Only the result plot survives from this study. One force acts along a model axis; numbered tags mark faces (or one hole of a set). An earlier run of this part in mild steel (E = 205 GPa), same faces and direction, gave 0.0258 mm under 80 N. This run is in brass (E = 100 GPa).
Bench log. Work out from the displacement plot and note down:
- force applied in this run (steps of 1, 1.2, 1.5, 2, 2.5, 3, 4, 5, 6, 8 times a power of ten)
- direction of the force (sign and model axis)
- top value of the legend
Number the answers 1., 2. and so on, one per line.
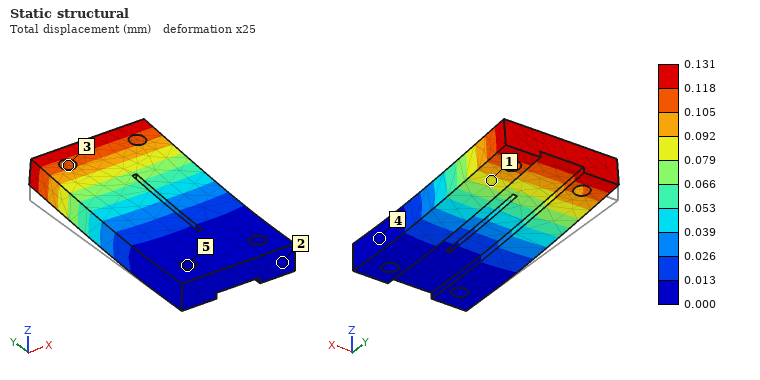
1. 200 N
2. +Z
3. 0.131 mm
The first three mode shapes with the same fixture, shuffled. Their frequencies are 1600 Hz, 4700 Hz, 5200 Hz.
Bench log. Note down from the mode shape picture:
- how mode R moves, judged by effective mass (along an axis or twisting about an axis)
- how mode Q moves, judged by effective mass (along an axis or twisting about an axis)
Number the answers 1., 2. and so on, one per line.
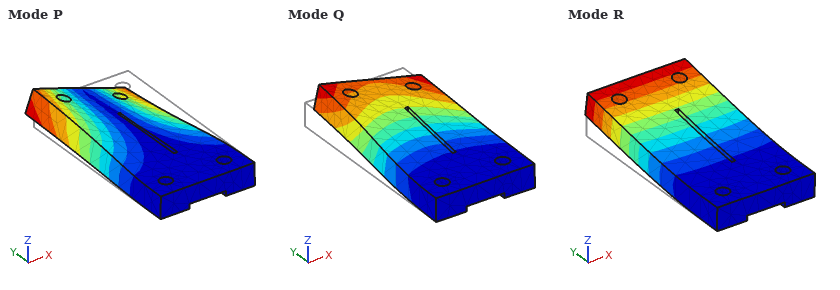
1. along Z
2. along X
